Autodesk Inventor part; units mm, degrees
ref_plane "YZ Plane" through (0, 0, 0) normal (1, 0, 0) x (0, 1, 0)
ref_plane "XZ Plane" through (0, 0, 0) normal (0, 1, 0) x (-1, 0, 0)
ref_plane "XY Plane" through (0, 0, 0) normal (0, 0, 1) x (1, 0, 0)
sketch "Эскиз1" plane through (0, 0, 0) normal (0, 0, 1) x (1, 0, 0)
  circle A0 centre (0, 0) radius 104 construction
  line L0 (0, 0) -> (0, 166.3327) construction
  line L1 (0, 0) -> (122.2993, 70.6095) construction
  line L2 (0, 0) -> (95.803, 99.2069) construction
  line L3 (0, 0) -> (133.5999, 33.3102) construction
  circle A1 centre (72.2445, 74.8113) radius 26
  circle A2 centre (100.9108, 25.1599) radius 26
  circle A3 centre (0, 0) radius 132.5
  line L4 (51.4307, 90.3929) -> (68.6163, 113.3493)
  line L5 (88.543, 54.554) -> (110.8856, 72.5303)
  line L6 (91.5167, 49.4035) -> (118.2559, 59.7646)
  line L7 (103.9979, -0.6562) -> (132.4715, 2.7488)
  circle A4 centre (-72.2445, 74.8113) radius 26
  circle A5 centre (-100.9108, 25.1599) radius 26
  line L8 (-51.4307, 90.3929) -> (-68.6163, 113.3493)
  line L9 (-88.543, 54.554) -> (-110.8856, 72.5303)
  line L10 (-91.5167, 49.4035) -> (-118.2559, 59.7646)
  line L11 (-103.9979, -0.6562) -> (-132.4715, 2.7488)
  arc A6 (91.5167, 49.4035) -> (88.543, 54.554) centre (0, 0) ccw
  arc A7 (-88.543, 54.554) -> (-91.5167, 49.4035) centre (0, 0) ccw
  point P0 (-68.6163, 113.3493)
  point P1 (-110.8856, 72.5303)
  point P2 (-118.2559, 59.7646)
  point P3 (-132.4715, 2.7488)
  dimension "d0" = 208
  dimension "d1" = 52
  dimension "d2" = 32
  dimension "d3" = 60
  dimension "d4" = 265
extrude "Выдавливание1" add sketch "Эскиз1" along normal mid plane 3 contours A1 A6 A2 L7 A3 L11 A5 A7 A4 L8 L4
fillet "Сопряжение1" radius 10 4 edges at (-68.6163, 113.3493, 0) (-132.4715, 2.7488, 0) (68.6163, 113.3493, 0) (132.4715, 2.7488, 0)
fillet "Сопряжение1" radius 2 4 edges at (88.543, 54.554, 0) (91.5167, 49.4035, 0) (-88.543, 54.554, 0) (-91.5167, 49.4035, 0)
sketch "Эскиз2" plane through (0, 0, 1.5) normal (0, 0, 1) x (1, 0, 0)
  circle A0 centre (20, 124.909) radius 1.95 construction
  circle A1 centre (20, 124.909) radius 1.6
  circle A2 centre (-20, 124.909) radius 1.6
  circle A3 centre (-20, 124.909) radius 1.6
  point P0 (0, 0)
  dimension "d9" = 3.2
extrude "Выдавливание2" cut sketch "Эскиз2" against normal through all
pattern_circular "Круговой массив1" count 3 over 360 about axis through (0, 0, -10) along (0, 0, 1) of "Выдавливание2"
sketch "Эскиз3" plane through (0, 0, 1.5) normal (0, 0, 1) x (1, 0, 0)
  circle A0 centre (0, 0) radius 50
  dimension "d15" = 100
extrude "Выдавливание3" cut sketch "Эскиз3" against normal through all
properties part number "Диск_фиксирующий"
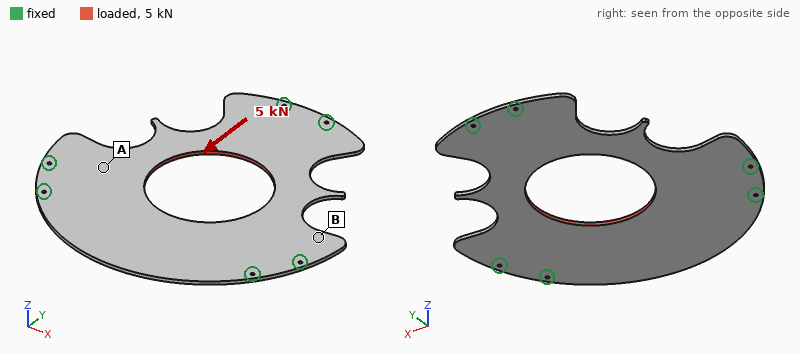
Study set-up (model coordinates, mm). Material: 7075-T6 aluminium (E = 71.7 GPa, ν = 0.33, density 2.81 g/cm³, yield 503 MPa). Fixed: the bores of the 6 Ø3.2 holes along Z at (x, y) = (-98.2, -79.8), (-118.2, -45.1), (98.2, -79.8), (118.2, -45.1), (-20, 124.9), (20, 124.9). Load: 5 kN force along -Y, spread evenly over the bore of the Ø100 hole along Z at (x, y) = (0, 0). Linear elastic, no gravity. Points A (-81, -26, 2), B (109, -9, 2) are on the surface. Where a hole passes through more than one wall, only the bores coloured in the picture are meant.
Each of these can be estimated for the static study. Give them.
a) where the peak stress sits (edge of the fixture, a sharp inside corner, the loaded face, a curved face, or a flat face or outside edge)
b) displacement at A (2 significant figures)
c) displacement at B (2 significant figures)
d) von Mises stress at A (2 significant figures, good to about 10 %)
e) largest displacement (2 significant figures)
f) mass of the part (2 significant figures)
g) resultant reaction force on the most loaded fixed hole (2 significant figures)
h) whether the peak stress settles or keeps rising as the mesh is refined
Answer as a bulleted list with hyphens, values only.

- edge of the fixture
- 17 µm
- 14 µm
- 6.0 MPa
- 32 µm
- 300 g
- 1.3 kN
- keeps rising
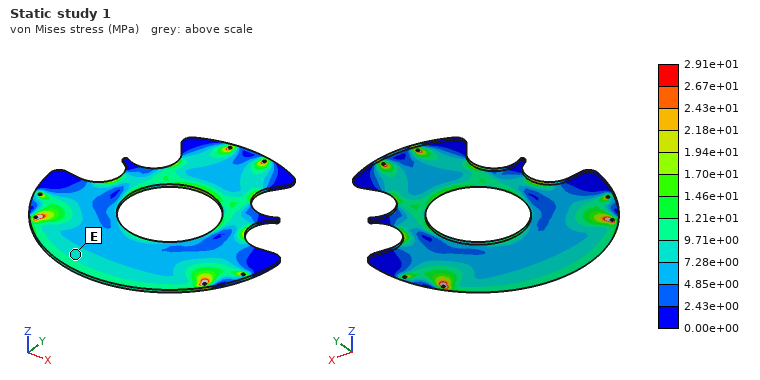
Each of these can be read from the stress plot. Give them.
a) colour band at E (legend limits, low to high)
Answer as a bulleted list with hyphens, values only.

- 7.28e+00 to 9.71e+00 MPa
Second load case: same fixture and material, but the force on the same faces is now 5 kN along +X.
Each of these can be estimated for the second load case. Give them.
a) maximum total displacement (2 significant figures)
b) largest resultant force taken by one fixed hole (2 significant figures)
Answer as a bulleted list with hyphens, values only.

- 50 µm
- 1.4 kN
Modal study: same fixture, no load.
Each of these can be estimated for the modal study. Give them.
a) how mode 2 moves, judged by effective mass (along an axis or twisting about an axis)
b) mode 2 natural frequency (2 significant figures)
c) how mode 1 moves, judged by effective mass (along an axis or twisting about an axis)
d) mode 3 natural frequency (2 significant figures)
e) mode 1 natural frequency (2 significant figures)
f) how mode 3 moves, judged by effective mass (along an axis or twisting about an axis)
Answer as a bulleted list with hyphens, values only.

- along Z
- 360 Hz
- along Z
- 490 Hz
- 320 Hz
- twisting about Y
